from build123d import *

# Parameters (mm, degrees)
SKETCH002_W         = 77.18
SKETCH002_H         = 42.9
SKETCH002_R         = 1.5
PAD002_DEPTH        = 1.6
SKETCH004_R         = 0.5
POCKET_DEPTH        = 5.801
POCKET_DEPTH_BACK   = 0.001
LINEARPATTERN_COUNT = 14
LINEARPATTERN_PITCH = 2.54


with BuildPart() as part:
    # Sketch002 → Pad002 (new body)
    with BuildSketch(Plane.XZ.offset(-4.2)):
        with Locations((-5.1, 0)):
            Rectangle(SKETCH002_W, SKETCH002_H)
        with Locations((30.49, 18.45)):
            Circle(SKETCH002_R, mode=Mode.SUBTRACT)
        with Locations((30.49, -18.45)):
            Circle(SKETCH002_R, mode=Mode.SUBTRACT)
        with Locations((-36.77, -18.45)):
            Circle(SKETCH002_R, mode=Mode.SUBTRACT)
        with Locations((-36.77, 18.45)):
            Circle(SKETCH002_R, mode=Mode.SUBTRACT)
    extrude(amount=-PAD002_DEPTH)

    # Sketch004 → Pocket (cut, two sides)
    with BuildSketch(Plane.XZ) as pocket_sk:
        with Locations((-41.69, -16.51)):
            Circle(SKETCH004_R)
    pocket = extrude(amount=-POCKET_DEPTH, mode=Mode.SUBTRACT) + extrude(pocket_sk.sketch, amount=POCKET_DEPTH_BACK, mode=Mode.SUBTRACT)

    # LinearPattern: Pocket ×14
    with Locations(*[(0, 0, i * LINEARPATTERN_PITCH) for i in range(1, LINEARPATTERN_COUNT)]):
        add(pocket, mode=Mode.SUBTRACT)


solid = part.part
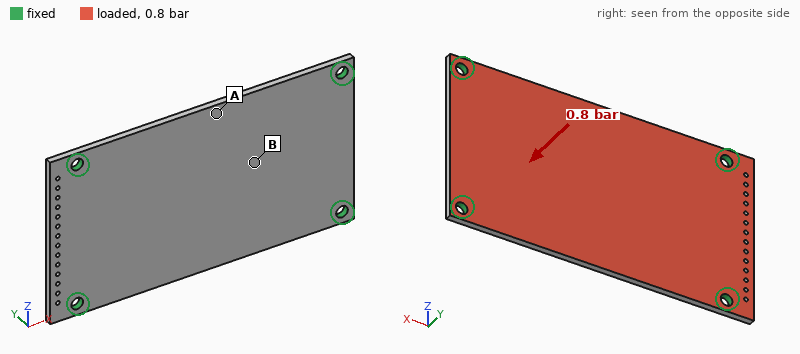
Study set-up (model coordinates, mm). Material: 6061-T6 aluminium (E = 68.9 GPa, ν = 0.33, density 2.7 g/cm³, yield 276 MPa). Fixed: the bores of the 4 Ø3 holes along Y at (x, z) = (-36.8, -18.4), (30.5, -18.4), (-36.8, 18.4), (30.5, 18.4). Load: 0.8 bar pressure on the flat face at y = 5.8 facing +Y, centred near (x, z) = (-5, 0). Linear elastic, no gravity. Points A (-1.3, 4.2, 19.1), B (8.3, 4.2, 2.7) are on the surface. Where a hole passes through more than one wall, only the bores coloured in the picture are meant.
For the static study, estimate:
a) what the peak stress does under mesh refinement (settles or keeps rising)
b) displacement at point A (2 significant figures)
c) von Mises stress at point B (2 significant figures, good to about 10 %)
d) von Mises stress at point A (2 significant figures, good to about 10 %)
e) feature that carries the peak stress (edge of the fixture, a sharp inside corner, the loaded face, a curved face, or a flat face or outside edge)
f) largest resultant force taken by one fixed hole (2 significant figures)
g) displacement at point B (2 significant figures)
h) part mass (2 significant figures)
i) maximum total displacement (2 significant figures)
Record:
keeps rising
0.23 mm
25 MPa
43 MPa
edge of the fixture
69 N
0.19 mm
14 g
0.23 mm
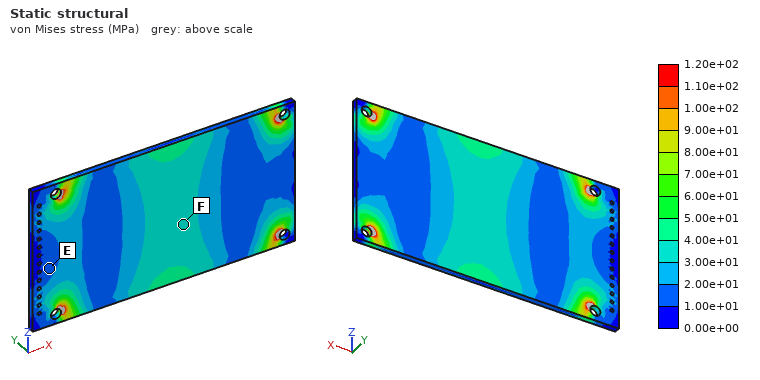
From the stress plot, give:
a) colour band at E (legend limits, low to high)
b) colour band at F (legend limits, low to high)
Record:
1.00e+01 to 2.00e+01 MPa
3.00e+01 to 4.00e+01 MPa
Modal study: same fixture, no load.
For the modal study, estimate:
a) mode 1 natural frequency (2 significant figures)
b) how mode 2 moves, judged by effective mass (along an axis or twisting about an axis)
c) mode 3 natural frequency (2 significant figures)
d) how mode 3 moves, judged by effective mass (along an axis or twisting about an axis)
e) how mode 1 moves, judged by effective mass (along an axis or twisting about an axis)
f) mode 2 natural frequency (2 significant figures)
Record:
1600 Hz
twisting about X
4400 Hz
twisting about Z
along Y
2700 Hz
